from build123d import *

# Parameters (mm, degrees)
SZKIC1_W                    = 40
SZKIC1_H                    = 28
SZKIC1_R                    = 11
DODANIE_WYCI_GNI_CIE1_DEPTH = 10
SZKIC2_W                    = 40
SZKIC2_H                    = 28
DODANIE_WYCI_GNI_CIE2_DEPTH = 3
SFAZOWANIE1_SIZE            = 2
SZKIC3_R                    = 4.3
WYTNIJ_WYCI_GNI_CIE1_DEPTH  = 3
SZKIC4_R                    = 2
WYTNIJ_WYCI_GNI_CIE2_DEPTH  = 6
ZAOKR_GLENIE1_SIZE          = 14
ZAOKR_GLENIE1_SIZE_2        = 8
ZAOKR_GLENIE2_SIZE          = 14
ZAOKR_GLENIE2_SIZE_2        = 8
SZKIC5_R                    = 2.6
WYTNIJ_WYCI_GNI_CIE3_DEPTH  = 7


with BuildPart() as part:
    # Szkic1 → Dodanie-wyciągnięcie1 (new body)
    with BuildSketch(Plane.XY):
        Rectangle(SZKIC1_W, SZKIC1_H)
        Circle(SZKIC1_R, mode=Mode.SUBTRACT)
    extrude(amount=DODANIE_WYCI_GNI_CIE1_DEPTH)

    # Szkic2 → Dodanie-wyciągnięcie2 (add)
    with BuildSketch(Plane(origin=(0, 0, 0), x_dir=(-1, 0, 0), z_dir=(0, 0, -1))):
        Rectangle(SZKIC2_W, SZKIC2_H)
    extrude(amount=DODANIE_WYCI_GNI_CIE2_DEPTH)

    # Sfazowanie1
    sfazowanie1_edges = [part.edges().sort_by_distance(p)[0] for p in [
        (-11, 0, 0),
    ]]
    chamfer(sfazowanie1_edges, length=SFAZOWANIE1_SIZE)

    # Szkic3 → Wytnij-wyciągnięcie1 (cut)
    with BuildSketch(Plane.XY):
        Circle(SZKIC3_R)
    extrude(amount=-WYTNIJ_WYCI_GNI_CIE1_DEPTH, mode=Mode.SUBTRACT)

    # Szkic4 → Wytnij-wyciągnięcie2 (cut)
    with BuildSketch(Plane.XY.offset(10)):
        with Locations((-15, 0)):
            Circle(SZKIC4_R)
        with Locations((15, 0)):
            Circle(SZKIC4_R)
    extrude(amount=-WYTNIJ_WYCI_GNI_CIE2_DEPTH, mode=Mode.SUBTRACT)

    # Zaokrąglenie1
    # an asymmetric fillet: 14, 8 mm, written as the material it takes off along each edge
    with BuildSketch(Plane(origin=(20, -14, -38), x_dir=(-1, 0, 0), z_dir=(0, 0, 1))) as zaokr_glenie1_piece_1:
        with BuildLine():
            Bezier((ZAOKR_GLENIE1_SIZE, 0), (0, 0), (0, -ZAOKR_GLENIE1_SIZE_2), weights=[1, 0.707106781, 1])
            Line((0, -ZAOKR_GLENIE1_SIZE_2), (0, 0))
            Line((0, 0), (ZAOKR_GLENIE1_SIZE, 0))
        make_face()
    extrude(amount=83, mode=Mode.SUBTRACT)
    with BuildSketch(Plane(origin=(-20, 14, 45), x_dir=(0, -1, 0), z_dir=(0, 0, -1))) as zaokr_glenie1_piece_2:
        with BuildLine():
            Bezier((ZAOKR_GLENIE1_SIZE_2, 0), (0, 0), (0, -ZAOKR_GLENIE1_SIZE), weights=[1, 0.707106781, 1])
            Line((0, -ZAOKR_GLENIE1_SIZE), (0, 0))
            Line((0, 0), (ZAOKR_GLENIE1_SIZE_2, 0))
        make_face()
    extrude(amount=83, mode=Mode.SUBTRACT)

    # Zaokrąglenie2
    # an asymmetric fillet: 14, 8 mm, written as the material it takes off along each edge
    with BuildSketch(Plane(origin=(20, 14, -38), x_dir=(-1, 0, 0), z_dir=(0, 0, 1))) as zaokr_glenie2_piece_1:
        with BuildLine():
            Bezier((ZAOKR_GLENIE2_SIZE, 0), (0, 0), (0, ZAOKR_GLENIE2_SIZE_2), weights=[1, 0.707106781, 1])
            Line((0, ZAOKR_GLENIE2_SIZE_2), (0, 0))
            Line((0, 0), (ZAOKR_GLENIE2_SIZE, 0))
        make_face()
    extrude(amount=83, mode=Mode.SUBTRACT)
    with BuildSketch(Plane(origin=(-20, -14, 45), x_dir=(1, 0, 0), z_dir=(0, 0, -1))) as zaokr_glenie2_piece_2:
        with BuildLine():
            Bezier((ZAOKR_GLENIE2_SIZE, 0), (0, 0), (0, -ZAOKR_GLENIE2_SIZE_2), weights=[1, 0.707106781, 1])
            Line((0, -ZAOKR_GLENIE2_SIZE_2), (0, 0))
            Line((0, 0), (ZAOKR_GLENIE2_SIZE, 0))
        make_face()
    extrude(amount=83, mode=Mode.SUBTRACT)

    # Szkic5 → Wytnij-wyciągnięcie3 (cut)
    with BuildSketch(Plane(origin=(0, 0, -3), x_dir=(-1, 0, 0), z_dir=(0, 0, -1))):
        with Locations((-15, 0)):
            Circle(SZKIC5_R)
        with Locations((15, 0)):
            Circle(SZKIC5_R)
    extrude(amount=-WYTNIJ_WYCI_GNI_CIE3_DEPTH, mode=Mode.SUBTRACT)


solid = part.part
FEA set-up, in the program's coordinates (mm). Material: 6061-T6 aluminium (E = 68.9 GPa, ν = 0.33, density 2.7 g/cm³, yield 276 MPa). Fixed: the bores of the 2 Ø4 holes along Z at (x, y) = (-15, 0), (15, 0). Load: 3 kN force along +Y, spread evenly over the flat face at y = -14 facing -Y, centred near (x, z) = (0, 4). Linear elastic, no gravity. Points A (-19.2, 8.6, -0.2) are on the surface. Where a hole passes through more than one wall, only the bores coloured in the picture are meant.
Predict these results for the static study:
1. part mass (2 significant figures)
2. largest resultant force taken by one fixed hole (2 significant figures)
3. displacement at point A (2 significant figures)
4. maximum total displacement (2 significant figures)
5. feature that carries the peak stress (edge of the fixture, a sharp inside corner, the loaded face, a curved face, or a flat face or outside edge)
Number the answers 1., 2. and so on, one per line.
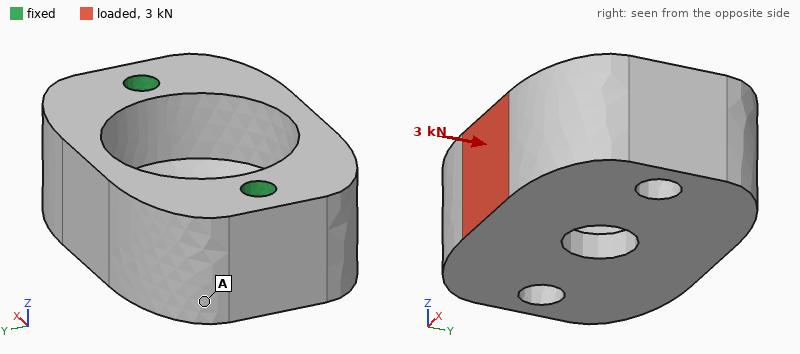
1. 24 g
2. 1.7 kN
3. 7.4 µm
4. 24 µm
5. edge of the fixture
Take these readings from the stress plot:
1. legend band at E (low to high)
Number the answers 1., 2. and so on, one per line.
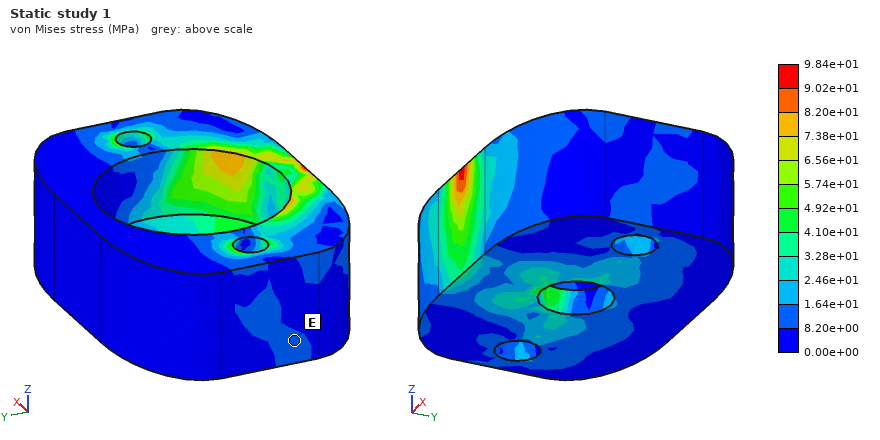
1. 8.20e+00 to 1.64e+01 MPa
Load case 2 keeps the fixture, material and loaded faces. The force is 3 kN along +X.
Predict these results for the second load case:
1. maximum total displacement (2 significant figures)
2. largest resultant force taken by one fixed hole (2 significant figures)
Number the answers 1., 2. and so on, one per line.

1. 18 µm
2. 1.9 kN
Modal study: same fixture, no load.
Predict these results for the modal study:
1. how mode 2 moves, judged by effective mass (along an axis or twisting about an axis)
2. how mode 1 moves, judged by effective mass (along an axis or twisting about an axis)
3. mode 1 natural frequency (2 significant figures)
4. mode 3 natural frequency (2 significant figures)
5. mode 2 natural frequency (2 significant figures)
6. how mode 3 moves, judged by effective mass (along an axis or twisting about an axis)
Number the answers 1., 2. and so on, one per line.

1. twisting about Z
2. along Y
3. 13 kHz
4. 24 kHz
5. 23 kHz
6. along Z
